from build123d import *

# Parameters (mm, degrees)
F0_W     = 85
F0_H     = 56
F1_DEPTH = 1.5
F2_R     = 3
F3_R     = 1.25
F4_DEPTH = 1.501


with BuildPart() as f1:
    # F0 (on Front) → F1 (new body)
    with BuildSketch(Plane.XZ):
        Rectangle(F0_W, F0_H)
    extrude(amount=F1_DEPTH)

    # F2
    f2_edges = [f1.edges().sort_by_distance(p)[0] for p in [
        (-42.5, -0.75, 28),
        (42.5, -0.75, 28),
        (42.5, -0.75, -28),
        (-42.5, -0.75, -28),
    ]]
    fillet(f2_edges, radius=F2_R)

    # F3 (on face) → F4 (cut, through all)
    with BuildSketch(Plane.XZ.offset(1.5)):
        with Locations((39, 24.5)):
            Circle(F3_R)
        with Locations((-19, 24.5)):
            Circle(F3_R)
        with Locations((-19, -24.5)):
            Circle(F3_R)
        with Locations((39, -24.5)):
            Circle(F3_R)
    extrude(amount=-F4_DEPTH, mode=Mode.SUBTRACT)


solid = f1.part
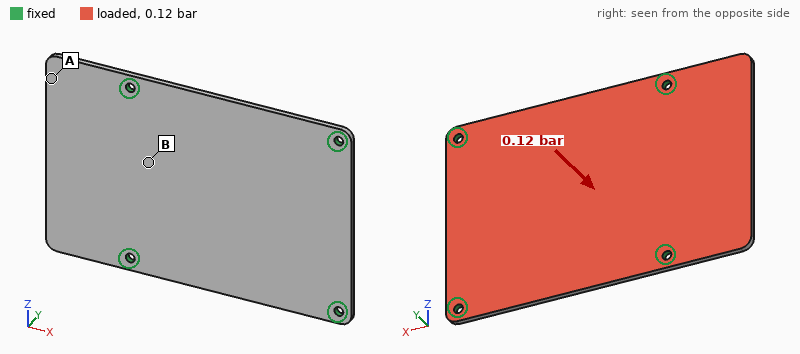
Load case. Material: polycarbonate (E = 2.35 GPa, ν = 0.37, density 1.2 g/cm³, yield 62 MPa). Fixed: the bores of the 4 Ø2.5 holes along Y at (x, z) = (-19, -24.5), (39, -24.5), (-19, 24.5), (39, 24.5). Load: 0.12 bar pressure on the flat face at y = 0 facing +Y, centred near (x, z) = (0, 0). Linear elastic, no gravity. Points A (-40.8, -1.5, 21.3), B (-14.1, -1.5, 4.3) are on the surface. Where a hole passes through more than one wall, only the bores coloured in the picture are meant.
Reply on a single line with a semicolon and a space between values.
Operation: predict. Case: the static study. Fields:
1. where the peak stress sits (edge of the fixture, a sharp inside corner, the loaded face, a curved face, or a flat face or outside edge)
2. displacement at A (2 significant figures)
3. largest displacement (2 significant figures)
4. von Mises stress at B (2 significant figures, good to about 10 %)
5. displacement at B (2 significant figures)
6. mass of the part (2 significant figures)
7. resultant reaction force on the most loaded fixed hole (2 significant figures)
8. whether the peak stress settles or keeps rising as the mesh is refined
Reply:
edge of the fixture; 0.69 mm; 1.1 mm; 5.3 MPa; 0.55 mm; 8.5 g; 18 N; keeps rising
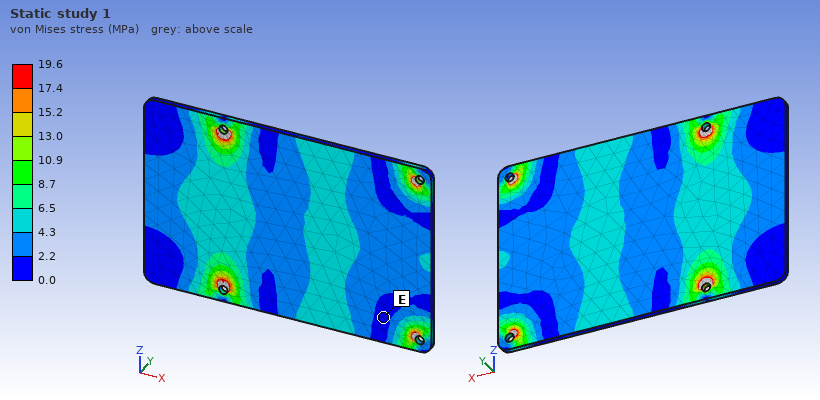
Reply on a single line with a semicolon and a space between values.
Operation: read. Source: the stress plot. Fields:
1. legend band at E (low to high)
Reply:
0.0 to 2.2 MPa
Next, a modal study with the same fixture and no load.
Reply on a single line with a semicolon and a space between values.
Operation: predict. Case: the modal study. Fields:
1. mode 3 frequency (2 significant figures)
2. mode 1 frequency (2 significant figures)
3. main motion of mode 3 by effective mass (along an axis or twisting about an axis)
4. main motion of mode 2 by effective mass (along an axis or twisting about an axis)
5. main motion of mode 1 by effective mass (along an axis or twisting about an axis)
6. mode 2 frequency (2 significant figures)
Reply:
770 Hz; 430 Hz; twisting about X; along Y; twisting about Z; 510 Hz
